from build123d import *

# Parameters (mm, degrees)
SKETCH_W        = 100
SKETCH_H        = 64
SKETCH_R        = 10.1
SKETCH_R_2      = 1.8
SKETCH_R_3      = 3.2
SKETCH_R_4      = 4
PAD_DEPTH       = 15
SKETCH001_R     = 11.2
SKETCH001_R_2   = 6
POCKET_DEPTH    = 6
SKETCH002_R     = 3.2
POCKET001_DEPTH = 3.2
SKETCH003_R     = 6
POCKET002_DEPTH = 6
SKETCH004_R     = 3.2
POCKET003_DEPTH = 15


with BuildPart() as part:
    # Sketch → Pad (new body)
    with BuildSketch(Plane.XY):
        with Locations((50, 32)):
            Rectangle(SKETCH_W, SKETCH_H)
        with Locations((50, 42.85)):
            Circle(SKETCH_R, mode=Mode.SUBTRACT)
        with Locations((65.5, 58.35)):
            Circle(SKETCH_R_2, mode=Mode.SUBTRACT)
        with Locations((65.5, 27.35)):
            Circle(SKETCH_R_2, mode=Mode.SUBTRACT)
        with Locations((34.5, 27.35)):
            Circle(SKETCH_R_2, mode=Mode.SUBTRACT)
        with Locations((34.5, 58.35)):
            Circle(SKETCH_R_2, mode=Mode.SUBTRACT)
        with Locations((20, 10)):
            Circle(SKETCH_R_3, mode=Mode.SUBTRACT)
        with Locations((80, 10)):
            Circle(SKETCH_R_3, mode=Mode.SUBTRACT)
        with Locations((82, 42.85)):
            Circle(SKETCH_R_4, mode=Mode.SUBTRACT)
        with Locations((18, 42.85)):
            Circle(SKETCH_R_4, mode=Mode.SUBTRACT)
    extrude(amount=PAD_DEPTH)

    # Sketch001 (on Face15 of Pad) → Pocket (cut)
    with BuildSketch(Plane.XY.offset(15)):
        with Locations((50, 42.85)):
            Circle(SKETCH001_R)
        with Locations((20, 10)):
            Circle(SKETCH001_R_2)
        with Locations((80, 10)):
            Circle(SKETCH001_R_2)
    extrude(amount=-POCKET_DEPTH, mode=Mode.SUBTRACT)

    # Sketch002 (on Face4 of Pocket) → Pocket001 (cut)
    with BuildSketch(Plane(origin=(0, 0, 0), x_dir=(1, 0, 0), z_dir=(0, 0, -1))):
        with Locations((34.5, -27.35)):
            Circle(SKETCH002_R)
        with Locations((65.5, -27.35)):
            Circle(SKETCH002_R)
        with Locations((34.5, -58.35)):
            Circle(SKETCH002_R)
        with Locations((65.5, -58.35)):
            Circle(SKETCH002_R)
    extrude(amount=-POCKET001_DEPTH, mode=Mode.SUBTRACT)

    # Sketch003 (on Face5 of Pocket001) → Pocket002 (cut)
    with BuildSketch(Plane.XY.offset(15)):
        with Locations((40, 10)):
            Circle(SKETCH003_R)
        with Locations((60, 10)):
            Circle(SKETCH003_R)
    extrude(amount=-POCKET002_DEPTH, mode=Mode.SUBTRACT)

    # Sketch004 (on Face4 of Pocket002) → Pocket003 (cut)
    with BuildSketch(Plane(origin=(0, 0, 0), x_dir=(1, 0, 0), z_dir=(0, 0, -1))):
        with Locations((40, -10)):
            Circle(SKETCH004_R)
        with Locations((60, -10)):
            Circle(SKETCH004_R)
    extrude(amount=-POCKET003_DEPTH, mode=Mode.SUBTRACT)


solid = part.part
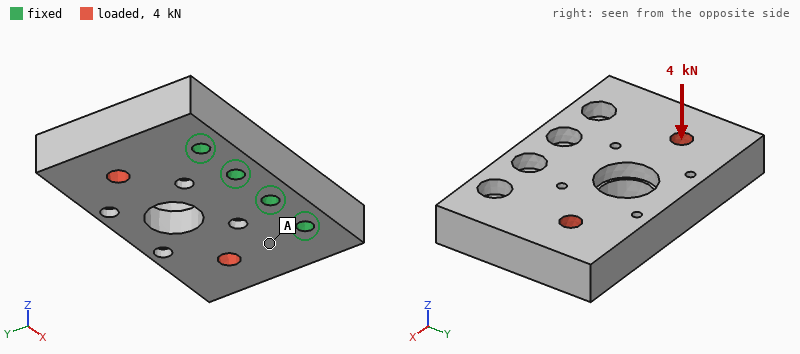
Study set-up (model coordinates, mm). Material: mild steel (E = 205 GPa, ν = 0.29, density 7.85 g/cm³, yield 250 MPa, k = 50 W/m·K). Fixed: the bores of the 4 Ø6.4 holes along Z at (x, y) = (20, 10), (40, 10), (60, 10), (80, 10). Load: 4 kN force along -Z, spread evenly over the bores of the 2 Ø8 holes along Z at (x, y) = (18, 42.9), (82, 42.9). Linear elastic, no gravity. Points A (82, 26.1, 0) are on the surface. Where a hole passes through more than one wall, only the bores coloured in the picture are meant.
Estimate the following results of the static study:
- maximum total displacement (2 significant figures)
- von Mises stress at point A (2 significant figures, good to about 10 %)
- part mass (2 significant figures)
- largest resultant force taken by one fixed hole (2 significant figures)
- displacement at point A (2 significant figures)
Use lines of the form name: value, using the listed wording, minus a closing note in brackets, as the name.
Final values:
maximum total displacement: 39 µm
von Mises stress at point A: 18 MPa
part mass: 660 g
largest resultant force taken by one fixed hole: 1.4 kN
displacement at point A: 9.5 µm
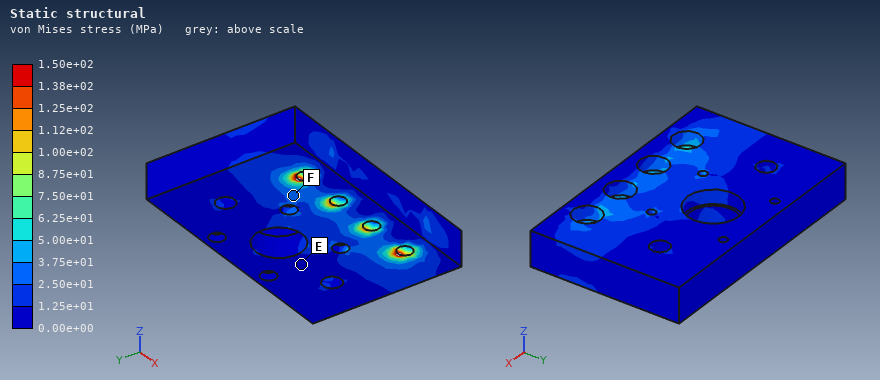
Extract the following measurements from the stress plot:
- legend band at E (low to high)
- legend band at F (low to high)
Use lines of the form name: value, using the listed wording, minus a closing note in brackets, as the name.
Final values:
legend band at E: 0.00e+00 to 1.25e+01 MPa
legend band at F: 2.50e+01 to 3.75e+01 MPa
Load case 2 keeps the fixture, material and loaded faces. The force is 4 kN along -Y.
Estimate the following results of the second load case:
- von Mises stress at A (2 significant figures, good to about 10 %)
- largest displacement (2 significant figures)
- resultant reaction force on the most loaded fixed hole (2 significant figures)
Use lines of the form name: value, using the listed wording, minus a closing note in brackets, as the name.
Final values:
von Mises stress at A: 5.4 MPa
largest displacement: 2.7 µm
resultant reaction force on the most loaded fixed hole: 1.4 kN
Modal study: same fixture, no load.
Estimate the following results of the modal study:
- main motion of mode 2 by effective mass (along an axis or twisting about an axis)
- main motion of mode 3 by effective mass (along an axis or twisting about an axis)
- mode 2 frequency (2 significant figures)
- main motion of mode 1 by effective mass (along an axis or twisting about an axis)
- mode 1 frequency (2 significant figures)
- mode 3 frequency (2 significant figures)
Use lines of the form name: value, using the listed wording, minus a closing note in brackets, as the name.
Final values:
main motion of mode 2 by effective mass: twisting about Y
main motion of mode 3 by effective mass: along X
mode 2 frequency: 4400 Hz
main motion of mode 1 by effective mass: along Z
mode 1 frequency: 2900 Hz
mode 3 frequency: 8200 Hz
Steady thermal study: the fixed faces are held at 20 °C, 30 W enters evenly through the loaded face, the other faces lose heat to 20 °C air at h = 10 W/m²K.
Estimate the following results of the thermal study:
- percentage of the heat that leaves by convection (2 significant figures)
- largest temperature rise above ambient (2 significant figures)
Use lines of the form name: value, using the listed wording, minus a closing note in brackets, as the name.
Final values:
percentage of the heat that leaves by convection: 6.3 %
largest temperature rise above ambient: 20 K
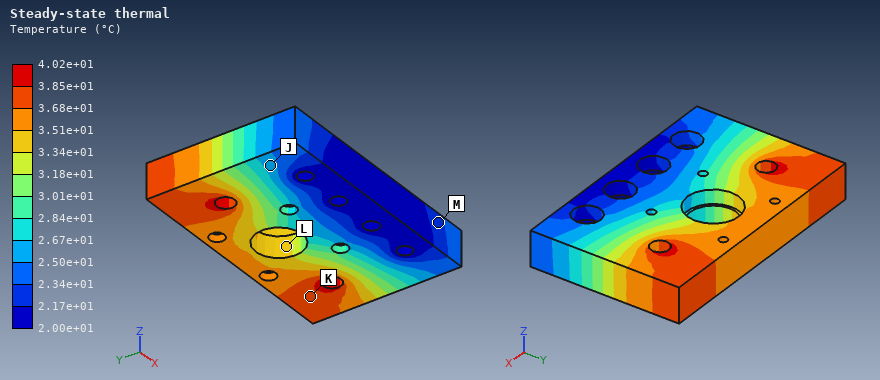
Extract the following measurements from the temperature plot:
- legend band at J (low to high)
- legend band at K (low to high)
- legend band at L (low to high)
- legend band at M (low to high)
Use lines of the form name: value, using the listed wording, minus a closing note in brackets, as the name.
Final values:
legend band at J: 2.50e+01 to 2.67e+01 °C
legend band at K: 3.68e+01 to 3.85e+01 °C
legend band at L: 3.34e+01 to 3.51e+01 °C
legend band at M: 2.17e+01 to 2.34e+01 °C
